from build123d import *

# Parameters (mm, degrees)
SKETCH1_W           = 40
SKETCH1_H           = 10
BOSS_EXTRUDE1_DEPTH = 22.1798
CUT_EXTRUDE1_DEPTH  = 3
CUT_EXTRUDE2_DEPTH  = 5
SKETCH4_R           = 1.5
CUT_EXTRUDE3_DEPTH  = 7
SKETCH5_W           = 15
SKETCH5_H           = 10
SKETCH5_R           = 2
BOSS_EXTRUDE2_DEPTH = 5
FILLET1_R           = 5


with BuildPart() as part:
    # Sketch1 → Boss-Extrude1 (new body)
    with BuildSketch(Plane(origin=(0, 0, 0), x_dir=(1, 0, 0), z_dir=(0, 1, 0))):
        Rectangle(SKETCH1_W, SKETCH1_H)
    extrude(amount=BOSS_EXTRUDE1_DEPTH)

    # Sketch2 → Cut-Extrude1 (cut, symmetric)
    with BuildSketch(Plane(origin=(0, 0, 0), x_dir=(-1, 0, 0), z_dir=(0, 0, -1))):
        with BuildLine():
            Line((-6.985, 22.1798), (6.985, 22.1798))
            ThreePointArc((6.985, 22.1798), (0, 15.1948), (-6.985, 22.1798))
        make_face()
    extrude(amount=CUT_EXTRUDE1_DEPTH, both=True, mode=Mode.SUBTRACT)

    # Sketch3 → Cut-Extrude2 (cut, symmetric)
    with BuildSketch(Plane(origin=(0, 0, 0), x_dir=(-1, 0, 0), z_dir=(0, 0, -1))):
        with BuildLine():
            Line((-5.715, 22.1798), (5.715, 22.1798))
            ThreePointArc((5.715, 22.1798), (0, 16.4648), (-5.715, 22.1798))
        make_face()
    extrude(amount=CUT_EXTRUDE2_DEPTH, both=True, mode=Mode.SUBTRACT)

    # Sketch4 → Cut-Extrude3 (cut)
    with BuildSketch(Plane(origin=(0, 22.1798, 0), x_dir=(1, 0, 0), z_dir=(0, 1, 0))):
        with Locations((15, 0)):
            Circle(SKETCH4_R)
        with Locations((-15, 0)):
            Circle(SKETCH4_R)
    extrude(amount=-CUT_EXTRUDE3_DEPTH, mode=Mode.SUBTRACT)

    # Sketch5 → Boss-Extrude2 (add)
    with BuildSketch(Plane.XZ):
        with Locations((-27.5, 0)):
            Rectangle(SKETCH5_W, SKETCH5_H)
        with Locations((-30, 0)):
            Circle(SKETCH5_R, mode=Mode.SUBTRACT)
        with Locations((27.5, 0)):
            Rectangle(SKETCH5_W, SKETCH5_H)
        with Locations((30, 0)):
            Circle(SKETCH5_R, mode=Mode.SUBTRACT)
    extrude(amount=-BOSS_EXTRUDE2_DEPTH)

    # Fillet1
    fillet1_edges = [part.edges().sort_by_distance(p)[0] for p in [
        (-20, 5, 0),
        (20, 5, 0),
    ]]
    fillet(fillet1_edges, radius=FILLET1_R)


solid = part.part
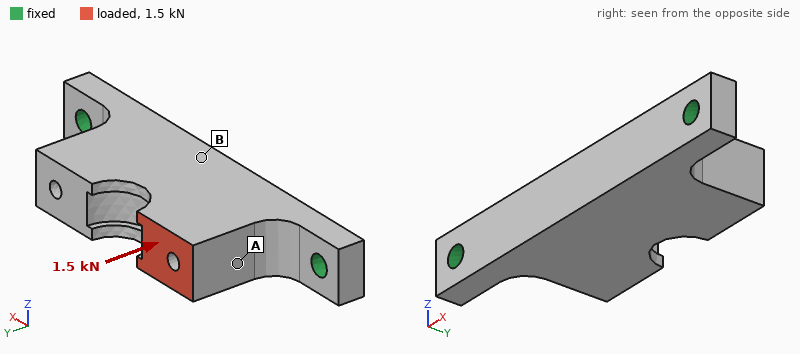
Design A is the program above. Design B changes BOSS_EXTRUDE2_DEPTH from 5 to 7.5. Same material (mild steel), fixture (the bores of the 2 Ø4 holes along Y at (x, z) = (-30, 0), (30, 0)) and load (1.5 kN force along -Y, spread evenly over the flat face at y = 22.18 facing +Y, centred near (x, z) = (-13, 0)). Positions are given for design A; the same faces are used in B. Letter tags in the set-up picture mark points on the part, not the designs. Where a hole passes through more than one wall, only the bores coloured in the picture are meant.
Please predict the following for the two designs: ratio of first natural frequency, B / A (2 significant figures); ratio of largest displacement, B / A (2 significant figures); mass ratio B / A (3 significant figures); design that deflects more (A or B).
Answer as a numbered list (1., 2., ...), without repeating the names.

1. 1.5
2. 0.60
3. 1.07
4. A
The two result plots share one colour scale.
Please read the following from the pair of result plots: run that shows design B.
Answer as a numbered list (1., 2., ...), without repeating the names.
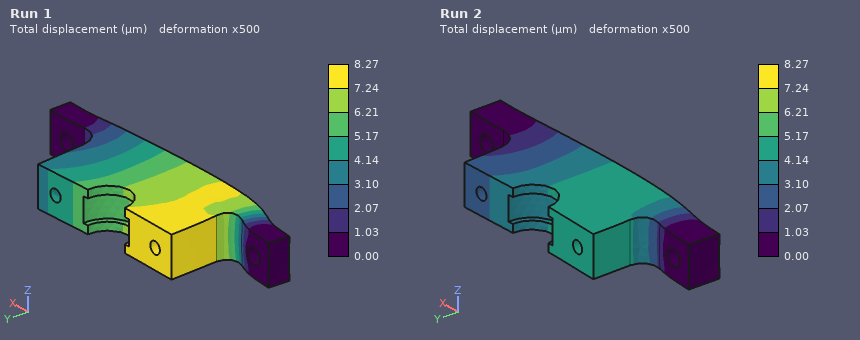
1. Run 2
